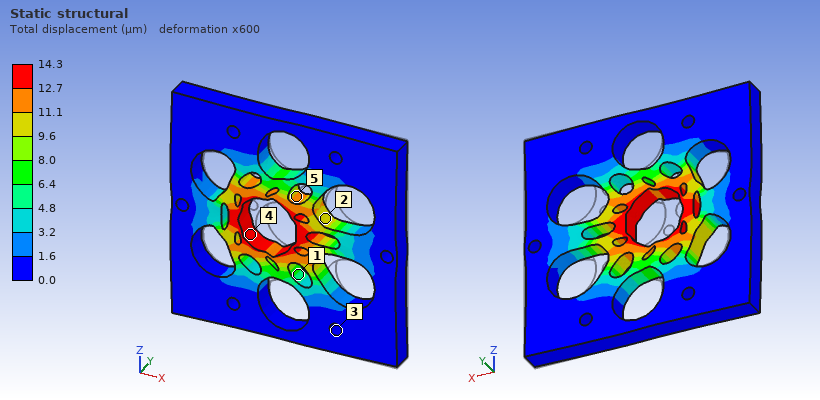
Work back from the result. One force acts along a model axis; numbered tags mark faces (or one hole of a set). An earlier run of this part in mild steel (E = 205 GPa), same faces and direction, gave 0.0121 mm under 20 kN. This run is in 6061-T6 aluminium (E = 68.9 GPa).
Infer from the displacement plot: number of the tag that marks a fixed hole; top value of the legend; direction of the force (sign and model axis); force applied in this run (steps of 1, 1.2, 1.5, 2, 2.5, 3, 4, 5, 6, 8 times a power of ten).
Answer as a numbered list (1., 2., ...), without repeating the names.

1. 3
2. 14.3 µm
3. -X
4. 8 kN
